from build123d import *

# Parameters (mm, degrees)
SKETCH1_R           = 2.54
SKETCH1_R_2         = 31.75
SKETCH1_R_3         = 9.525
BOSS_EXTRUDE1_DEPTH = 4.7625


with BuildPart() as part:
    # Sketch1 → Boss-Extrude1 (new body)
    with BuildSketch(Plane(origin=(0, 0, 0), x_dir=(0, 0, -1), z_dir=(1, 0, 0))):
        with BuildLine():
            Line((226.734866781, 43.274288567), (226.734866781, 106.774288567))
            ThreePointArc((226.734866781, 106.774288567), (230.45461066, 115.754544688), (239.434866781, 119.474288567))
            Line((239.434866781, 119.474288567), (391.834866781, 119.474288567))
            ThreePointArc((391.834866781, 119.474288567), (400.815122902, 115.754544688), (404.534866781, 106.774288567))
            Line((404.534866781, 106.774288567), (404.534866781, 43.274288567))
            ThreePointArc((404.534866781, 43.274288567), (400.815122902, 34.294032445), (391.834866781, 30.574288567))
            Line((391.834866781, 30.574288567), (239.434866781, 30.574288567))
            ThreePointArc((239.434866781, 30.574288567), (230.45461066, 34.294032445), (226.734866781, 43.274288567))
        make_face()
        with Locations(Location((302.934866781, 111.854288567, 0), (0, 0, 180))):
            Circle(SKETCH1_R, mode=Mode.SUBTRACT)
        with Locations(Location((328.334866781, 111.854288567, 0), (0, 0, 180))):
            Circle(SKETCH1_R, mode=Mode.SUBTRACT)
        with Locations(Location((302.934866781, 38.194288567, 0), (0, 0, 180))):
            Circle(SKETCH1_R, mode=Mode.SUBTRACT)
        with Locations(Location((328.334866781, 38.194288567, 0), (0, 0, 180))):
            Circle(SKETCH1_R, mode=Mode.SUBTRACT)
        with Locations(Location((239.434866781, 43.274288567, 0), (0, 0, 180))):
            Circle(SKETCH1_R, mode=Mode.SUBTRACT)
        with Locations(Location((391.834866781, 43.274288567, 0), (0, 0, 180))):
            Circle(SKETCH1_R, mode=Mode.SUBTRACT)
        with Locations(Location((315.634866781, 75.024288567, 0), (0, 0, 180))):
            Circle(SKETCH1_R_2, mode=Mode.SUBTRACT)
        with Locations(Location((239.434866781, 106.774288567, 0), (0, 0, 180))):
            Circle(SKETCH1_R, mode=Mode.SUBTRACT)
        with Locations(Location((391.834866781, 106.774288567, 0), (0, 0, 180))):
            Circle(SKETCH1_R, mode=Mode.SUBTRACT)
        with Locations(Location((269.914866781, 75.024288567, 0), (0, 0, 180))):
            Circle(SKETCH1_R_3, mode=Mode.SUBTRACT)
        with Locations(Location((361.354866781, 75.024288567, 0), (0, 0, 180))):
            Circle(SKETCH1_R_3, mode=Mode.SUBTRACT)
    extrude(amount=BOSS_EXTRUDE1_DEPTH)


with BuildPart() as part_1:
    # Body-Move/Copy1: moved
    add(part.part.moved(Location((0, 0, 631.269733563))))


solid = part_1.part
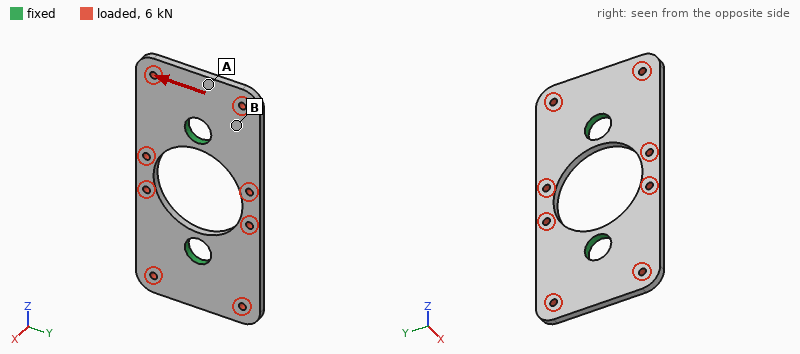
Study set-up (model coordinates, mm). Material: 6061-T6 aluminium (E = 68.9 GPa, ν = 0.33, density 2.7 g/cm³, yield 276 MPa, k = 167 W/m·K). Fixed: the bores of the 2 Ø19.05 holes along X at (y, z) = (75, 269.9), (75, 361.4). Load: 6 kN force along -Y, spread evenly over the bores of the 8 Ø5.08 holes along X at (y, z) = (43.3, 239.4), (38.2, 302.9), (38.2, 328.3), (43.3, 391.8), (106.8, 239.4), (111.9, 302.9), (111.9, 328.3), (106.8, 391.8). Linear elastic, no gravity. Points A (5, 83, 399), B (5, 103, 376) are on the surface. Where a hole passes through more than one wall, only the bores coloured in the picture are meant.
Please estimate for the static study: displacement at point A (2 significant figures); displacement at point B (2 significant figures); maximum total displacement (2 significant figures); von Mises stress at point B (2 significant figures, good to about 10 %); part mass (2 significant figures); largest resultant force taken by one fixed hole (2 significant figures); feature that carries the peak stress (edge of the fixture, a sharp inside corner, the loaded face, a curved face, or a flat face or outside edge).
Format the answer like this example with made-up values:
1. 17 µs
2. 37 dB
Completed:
1. 7.2 µm
2. 3.9 µm
3. 18 µm
4. 6.6 MPa
5. 150 g
6. 3.0 kN
7. the loaded face
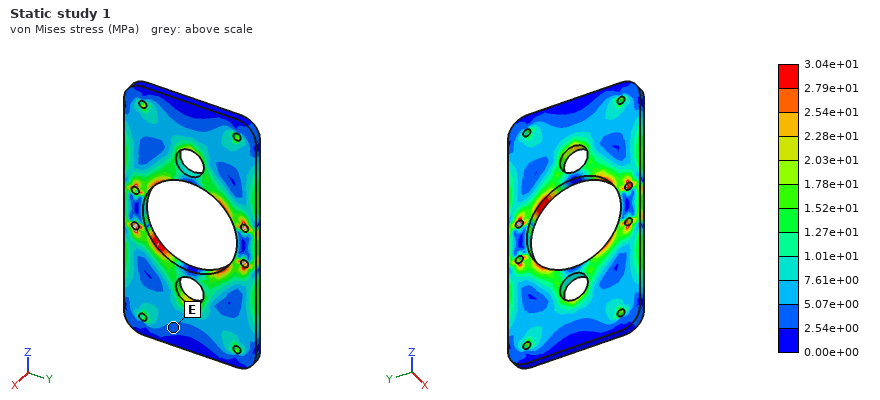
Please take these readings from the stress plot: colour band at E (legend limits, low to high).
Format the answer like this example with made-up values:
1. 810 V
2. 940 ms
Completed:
1. 2.54e+00 to 5.07e+00 MPa
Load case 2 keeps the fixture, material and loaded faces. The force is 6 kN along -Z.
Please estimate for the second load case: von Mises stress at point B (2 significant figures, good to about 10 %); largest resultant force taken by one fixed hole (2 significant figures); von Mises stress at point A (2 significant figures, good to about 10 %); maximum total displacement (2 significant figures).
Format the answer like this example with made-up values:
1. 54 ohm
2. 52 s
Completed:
1. 8.5 MPa
2. 3.0 kN
3. 9.1 MPa
4. 14 µm
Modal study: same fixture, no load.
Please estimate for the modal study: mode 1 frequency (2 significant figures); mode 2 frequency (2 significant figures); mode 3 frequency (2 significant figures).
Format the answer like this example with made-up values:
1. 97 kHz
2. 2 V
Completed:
1. 2000 Hz
2. 2000 Hz
3. 2200 Hz
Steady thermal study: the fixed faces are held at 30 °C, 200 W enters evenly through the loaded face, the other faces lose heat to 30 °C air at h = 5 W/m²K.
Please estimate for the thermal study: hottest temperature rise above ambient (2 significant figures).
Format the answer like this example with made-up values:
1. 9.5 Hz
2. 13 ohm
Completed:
1. 72 K
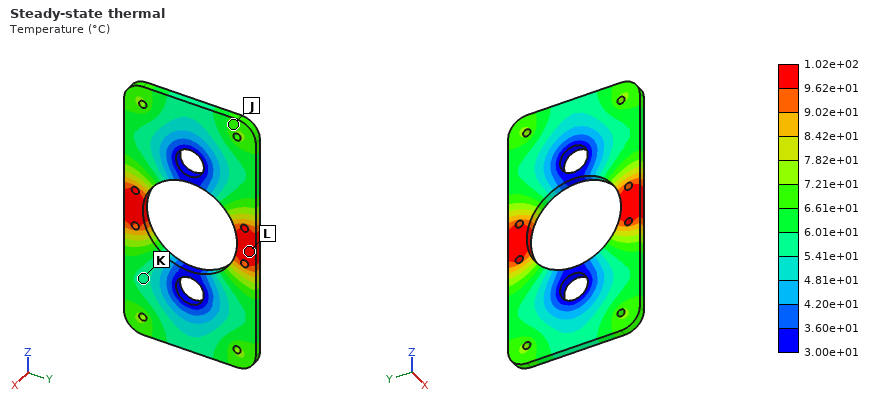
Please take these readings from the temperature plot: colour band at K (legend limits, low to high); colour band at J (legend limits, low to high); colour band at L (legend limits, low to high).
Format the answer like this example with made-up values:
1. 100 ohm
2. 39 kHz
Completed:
1. 5.41e+01 to 6.01e+01 °C
2. 6.61e+01 to 7.21e+01 °C
3. 9.62e+01 to 1.02e+02 °C
